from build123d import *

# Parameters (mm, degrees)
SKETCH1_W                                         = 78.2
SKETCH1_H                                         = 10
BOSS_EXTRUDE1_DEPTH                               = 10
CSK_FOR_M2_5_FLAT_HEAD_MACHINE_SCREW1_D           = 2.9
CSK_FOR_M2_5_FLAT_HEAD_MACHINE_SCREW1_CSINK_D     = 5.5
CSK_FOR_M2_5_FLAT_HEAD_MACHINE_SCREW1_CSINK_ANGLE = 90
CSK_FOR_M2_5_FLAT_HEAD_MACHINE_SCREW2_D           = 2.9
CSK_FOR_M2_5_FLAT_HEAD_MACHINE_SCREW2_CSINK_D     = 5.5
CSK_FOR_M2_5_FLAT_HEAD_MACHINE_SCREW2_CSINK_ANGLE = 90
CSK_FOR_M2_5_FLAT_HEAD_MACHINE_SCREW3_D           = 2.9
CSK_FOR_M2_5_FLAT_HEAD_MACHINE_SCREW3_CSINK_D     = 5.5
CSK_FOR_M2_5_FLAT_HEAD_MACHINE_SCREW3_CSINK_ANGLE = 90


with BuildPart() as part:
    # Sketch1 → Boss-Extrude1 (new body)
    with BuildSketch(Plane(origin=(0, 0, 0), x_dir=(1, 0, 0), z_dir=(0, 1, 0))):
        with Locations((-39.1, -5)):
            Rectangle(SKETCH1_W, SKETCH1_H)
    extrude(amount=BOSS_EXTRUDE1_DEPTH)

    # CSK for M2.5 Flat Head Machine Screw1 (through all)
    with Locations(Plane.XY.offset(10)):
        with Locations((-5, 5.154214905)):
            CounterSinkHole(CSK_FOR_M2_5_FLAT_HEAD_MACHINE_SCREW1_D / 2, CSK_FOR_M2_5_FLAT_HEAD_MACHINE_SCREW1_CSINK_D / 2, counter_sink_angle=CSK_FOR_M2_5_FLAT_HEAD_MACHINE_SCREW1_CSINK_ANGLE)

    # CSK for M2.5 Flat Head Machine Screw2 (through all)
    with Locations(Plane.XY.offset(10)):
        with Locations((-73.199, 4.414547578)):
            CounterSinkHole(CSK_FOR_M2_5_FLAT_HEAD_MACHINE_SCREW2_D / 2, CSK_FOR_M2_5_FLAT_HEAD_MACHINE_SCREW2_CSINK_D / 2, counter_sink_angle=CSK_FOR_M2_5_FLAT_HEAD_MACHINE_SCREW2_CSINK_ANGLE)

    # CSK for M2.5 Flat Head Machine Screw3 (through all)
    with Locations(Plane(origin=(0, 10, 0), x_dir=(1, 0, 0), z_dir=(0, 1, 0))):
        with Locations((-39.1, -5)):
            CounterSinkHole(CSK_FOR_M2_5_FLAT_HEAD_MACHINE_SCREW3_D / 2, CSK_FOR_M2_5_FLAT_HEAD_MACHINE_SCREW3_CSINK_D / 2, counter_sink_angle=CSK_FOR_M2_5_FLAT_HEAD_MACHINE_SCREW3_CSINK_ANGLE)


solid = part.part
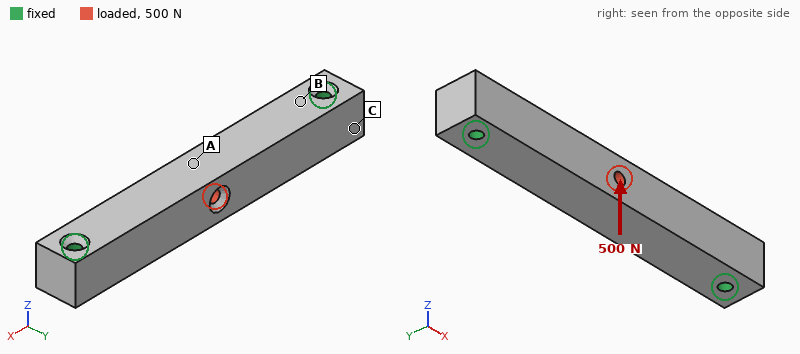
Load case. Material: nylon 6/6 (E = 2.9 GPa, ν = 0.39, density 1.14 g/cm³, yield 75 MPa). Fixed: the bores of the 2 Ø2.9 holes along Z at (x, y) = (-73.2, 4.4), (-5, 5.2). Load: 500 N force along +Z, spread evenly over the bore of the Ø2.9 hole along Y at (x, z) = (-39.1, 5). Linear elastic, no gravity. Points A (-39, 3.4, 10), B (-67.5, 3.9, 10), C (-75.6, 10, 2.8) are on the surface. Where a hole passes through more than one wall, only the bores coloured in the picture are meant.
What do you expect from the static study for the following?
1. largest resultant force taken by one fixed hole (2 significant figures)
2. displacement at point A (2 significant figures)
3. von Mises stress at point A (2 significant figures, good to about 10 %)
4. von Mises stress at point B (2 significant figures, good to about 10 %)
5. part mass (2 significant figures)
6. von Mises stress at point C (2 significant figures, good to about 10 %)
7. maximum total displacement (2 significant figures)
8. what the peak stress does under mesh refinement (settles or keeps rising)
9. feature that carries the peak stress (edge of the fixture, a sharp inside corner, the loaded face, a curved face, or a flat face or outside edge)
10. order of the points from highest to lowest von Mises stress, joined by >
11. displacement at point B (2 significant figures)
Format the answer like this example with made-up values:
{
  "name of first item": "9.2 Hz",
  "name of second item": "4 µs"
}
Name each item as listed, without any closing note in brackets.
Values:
{
  "largest resultant force taken by one fixed hole": "250 N",
  "displacement at point A": "0.47 mm",
  "von Mises stress at point A": "28 MPa",
  "von Mises stress at point B": "16 MPa",
  "part mass": "8.7 g",
  "von Mises stress at point C": "4.6 MPa",
  "maximum total displacement": "0.50 mm",
  "what the peak stress does under mesh refinement": "keeps rising",
  "feature that carries the peak stress": "edge of the fixture",
  "order of the points from highest to lowest von Mises stress, joined by >": "A > B > C",
  "displacement at point B": "0.080 mm"
}
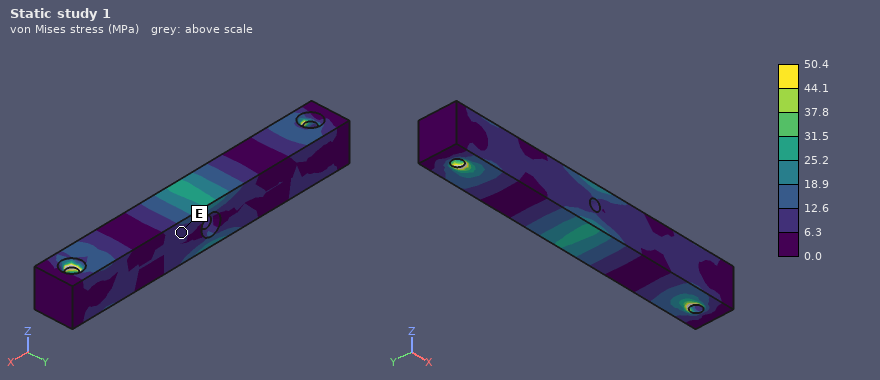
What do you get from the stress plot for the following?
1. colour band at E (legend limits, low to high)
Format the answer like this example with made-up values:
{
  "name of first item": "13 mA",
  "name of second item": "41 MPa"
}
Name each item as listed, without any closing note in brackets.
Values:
{
  "colour band at E": "6.3 to 12.6 MPa"
}
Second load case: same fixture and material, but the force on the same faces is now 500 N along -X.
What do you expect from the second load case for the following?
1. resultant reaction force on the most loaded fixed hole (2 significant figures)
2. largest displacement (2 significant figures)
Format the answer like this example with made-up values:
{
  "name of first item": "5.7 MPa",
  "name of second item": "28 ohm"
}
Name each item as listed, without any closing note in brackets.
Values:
{
  "resultant reaction force on the most loaded fixed hole": "250 N",
  "largest displacement": "37 µm"
}
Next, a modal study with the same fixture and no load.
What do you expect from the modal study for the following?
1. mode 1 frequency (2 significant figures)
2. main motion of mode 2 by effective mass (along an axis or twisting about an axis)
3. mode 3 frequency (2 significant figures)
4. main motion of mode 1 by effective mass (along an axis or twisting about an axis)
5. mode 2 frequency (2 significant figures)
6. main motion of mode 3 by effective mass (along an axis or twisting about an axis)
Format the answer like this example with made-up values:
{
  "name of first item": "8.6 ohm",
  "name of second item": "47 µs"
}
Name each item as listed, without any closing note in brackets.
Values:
{
  "mode 1 frequency": "2400 Hz",
  "main motion of mode 2 by effective mass": "along Z",
  "mode 3 frequency": "6400 Hz",
  "main motion of mode 1 by effective mass": "along Y",
  "mode 2 frequency": "3000 Hz",
  "main motion of mode 3 by effective mass": "twisting about X"
}
